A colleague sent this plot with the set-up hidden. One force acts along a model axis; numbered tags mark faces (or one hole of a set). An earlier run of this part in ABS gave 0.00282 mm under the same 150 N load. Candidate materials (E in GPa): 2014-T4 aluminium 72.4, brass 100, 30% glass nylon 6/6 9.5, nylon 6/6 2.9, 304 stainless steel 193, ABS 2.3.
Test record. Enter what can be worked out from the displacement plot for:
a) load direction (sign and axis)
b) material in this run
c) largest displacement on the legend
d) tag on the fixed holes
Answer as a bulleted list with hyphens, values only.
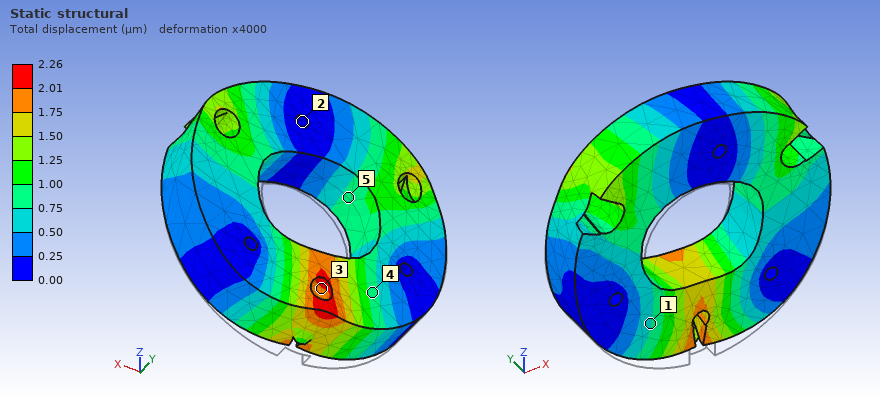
- +Z
- nylon 6/6
- 2.26 µm
- 2
